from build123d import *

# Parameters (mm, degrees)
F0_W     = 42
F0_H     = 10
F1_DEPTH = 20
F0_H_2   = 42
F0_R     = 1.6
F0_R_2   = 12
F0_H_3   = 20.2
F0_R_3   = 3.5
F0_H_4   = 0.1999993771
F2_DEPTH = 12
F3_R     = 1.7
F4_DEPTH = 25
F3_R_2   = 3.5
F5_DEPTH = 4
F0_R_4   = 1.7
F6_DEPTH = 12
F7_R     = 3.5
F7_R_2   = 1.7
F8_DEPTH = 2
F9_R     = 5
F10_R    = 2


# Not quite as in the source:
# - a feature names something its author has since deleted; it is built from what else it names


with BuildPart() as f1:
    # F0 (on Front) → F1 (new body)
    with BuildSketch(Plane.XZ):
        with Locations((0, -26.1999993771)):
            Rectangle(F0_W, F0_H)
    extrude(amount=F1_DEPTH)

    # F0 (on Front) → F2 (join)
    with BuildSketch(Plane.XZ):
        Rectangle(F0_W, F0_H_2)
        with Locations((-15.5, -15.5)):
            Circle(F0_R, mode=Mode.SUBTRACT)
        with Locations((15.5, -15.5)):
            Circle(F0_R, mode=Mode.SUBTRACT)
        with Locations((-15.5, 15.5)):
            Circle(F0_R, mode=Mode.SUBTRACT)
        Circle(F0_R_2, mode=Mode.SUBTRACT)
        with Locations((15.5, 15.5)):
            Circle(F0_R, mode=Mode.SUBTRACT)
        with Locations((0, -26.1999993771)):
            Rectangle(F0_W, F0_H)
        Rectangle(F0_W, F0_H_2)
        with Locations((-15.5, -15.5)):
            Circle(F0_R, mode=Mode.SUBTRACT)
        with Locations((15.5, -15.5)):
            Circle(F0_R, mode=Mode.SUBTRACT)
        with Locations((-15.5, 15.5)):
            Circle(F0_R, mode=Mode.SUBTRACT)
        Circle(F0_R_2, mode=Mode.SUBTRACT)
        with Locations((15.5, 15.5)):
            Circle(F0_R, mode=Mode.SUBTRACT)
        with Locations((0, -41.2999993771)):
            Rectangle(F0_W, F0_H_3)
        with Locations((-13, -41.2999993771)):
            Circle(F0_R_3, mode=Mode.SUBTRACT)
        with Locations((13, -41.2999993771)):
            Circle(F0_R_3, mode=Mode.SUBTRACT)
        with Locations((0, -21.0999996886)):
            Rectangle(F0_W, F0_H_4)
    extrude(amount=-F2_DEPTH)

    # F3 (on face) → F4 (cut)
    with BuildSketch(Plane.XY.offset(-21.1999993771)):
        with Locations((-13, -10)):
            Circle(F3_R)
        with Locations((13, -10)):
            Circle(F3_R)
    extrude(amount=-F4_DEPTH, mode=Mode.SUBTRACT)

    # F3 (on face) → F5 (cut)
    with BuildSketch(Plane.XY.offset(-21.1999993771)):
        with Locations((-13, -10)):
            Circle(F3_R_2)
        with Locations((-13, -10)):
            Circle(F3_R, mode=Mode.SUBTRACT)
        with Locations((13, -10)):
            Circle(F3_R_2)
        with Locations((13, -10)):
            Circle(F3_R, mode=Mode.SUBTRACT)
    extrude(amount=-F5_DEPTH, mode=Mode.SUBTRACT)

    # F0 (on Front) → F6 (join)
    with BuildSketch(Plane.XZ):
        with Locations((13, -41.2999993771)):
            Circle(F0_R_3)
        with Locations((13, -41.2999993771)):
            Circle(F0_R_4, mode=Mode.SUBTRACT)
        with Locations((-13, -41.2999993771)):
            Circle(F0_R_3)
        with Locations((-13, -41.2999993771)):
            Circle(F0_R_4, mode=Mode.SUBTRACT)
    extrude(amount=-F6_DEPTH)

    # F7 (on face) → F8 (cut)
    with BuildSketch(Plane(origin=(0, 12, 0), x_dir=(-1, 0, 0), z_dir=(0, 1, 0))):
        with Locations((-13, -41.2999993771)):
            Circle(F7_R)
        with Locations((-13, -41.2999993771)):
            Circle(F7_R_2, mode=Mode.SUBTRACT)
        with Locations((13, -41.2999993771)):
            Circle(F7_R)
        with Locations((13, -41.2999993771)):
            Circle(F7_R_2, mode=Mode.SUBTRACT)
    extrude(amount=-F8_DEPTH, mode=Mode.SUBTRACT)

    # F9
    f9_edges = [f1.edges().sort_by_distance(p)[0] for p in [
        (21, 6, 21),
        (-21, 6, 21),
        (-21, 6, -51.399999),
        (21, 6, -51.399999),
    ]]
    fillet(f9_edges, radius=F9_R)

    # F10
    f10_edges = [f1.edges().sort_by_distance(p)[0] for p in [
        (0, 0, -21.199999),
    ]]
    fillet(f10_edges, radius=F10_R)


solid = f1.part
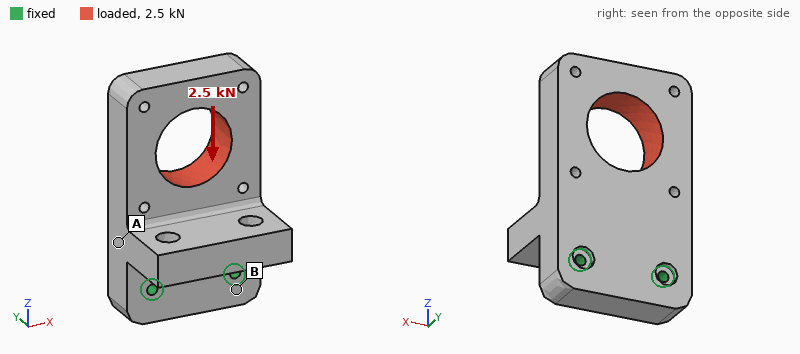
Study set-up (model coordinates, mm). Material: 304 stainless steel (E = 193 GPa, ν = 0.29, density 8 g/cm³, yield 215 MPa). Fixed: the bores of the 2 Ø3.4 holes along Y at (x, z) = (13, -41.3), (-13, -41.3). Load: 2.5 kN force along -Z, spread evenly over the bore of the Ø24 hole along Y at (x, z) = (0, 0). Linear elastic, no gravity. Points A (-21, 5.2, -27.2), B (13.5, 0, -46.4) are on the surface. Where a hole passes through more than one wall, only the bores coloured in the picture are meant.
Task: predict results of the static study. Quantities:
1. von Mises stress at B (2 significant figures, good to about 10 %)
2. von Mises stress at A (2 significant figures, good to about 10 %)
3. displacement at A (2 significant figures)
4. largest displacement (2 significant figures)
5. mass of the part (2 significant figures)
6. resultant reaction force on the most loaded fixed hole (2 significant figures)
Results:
2.2 MPa
7.3 MPa
0.66 µm
3.6 µm
300 g
1.3 kN
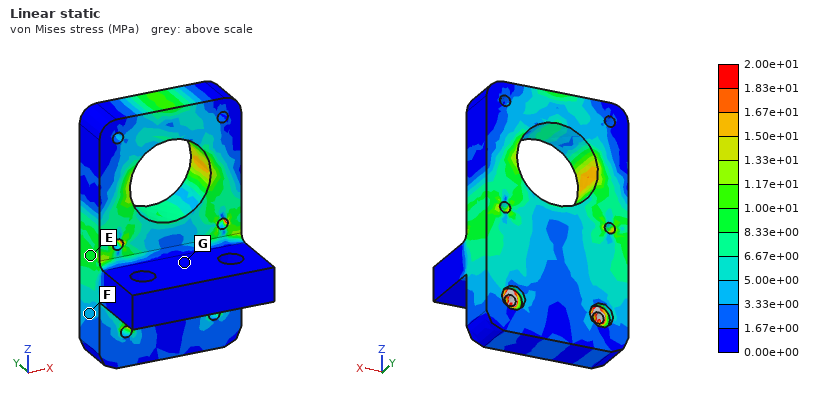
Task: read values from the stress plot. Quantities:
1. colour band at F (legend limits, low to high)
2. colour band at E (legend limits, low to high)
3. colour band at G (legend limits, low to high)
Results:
3.33e+00 to 5.00e+00 MPa
8.33e+00 to 1.00e+01 MPa
0.00e+00 to 1.67e+00 MPa
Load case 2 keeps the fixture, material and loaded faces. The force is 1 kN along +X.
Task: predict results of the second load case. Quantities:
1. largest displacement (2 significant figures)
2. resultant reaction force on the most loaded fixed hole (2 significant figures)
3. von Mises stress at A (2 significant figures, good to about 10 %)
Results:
8.0 µm
1.6 kN
8.1 MPa
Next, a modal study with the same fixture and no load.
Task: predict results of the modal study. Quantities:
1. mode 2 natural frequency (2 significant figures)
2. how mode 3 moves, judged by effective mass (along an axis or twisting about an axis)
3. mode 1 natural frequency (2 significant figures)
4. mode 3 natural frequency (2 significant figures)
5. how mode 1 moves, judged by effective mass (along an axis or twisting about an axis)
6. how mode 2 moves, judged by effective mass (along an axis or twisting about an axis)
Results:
5700 Hz
twisting about Z
2200 Hz
6200 Hz
along Y
along X
